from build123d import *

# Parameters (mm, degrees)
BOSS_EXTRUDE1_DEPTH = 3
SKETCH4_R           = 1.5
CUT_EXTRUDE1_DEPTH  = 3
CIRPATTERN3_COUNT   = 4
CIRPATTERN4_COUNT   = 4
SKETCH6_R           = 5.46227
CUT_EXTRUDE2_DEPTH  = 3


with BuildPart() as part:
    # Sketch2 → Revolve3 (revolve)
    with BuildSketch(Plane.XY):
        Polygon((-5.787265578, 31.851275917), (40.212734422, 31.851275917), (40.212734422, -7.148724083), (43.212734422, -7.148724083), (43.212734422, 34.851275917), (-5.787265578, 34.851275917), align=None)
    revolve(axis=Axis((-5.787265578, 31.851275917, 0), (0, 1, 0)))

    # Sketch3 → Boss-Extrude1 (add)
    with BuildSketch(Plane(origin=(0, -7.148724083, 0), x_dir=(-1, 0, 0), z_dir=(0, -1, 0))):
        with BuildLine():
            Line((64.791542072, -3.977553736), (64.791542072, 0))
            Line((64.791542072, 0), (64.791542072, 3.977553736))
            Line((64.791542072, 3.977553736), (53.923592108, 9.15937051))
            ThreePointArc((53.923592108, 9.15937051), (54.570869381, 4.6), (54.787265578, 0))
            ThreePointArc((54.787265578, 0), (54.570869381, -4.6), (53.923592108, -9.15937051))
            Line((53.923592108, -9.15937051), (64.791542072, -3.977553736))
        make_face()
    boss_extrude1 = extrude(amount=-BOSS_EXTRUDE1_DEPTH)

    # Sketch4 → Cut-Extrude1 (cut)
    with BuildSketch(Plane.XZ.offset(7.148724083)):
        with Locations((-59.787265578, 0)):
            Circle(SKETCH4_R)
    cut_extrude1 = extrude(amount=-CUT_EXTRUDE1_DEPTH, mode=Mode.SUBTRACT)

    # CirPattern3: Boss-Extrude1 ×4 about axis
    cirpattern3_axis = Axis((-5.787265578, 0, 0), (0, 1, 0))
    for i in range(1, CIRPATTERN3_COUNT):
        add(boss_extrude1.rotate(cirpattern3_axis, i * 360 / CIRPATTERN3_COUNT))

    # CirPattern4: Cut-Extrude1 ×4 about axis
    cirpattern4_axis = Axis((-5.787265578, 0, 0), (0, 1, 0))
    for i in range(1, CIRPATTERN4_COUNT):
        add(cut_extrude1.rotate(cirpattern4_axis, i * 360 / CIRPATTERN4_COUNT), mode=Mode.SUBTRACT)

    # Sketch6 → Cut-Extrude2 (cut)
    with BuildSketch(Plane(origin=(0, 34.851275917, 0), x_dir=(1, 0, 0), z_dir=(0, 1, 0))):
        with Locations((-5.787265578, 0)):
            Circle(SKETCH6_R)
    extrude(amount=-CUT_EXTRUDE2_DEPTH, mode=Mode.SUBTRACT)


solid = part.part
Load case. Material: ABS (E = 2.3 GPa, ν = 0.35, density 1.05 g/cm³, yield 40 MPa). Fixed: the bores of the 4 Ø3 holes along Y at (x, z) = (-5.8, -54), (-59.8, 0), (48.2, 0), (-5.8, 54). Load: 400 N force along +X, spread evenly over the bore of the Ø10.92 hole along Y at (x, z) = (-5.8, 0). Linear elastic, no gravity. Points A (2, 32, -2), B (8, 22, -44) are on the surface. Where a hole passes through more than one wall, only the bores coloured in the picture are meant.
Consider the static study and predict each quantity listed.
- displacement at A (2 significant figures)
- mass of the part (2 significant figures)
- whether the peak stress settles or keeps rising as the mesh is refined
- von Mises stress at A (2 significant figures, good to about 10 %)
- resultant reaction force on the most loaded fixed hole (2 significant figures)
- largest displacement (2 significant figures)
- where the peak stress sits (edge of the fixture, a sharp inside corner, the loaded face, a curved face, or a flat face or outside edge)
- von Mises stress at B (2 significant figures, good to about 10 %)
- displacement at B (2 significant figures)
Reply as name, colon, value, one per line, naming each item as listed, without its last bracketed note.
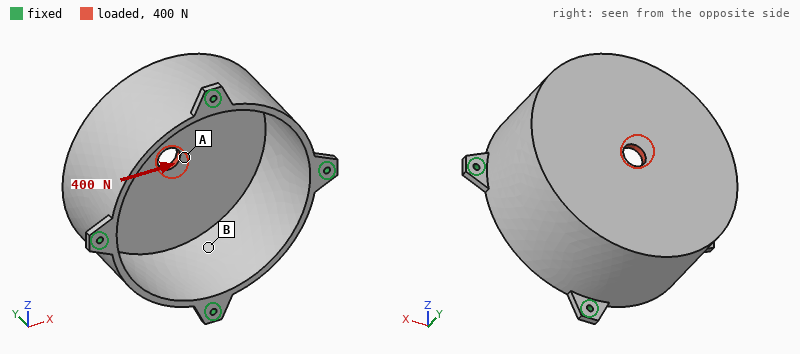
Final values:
displacement at A: 0.25 mm
mass of the part: 62 g
whether the peak stress settles or keeps rising as the mesh is refined: keeps rising
von Mises stress at A: 3.8 MPa
resultant reaction force on the most loaded fixed hole: 170 N
largest displacement: 0.26 mm
where the peak stress sits: edge of the fixture
von Mises stress at B: 1.3 MPa
displacement at B: 0.16 mm
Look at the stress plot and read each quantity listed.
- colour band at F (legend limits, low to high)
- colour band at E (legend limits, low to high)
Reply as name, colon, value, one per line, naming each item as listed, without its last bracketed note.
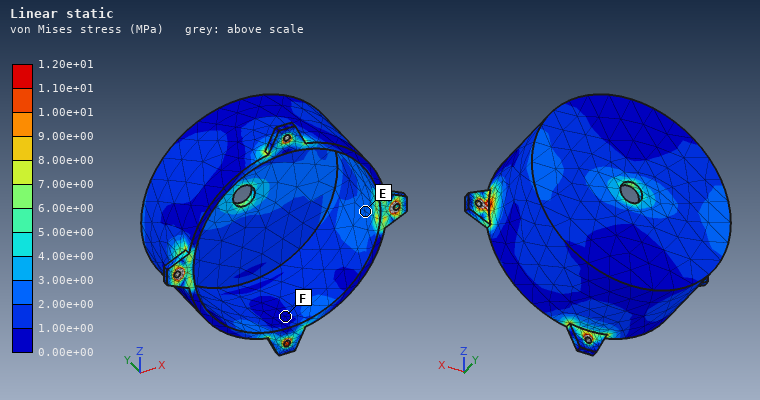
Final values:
colour band at F: 0.00e+00 to 1.00e+00 MPa
colour band at E: 2.00e+00 to 3.00e+00 MPa
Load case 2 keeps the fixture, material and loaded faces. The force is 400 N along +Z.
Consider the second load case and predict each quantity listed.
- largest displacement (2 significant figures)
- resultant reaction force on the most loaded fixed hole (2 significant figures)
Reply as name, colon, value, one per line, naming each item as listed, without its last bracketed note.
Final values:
largest displacement: 0.26 mm
resultant reaction force on the most loaded fixed hole: 170 N
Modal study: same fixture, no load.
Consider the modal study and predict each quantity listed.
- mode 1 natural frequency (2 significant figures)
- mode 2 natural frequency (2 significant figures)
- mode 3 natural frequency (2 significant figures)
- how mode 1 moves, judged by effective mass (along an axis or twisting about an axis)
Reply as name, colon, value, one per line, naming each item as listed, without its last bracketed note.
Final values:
mode 1 natural frequency: 820 Hz
mode 2 natural frequency: 1000 Hz
mode 3 natural frequency: 1000 Hz
how mode 1 moves, judged by effective mass: along Y
